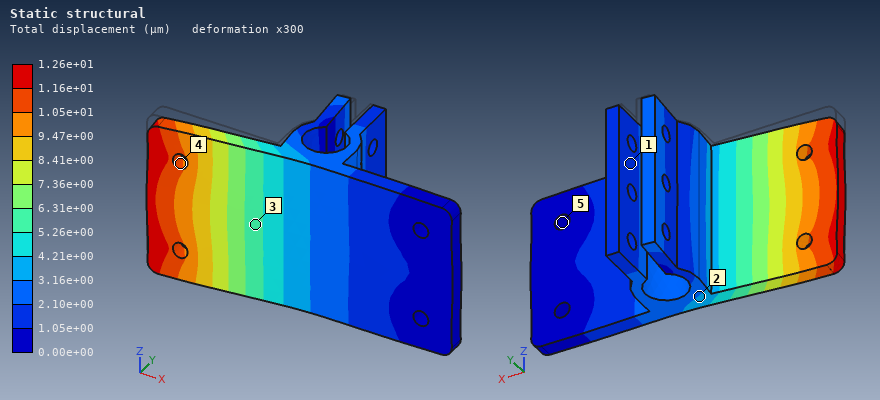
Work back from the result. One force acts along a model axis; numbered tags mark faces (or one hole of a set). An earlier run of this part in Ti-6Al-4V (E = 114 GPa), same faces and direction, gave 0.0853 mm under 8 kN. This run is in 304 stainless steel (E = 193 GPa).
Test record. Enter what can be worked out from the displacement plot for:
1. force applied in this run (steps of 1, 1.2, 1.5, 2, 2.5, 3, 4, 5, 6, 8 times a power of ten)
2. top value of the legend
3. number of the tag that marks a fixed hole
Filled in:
2 kN
1.26e+01 µm
5
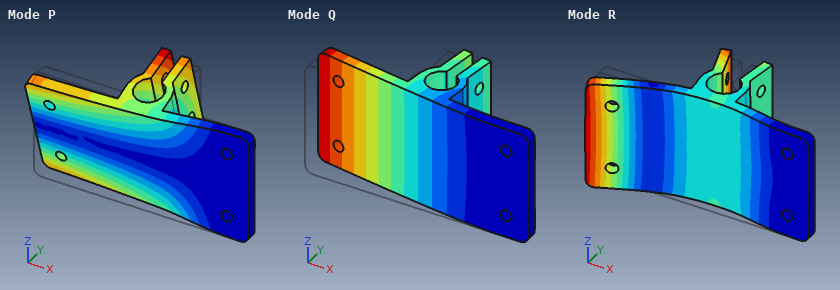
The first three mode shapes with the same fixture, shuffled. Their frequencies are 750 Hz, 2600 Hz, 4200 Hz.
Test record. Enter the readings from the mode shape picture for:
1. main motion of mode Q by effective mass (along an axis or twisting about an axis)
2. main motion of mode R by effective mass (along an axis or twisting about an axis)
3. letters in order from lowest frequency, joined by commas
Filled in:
along Y
along Y
Q, P, R
